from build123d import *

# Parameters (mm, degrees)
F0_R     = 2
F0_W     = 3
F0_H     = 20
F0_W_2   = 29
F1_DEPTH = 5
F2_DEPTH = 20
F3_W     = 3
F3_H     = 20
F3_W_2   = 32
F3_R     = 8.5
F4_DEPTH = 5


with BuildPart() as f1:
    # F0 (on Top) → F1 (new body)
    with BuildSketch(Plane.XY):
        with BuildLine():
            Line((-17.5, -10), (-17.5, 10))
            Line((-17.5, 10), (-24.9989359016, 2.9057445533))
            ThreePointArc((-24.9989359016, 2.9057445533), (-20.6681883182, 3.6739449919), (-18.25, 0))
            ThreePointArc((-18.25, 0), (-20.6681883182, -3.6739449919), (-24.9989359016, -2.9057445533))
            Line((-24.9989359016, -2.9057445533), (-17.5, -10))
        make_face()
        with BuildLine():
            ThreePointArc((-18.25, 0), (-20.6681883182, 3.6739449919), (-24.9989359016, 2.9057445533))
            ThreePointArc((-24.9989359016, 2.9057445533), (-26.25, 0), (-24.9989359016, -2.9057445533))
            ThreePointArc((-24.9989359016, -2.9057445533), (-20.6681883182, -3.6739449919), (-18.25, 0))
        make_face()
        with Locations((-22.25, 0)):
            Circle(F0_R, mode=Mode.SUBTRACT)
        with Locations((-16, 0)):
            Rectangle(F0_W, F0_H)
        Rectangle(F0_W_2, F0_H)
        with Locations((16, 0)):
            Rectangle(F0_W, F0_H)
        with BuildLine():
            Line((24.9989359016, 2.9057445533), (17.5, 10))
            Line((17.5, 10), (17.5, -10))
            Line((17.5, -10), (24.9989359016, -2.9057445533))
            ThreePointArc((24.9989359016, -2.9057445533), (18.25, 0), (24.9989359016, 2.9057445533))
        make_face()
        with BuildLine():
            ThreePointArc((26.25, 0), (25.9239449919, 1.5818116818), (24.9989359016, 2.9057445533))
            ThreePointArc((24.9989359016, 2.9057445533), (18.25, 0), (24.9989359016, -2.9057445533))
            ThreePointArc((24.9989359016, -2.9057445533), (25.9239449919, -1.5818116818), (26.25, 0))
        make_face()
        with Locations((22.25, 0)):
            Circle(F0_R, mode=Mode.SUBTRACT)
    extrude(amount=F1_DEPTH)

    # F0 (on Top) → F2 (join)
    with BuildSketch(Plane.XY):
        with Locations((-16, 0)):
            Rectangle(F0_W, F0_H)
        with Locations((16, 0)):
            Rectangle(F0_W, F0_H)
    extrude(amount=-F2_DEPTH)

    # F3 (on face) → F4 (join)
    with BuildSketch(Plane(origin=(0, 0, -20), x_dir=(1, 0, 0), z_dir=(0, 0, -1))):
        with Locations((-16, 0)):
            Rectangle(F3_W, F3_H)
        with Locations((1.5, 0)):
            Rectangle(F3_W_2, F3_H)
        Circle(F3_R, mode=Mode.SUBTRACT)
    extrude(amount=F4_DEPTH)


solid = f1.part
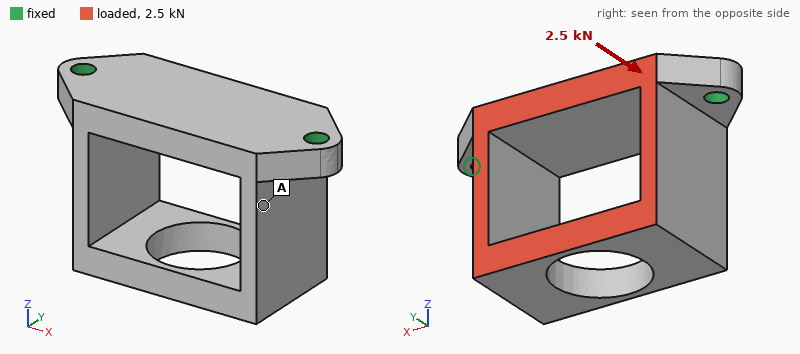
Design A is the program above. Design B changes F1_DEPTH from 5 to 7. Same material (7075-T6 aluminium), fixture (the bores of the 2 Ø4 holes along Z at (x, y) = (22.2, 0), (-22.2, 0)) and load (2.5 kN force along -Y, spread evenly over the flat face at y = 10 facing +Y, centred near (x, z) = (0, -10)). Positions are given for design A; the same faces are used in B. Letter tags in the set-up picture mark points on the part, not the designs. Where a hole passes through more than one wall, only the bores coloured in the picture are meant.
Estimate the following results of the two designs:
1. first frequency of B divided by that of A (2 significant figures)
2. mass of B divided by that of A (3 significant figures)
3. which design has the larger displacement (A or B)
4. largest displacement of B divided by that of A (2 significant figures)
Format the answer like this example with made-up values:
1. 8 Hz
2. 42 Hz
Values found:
1. 1.0
2. 1.19
3. A
4. 0.55
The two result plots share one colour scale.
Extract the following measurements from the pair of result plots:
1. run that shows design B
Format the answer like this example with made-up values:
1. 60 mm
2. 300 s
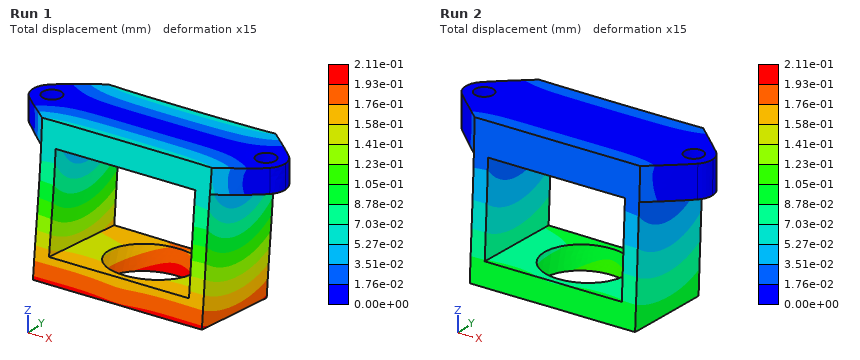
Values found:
1. Run 2
